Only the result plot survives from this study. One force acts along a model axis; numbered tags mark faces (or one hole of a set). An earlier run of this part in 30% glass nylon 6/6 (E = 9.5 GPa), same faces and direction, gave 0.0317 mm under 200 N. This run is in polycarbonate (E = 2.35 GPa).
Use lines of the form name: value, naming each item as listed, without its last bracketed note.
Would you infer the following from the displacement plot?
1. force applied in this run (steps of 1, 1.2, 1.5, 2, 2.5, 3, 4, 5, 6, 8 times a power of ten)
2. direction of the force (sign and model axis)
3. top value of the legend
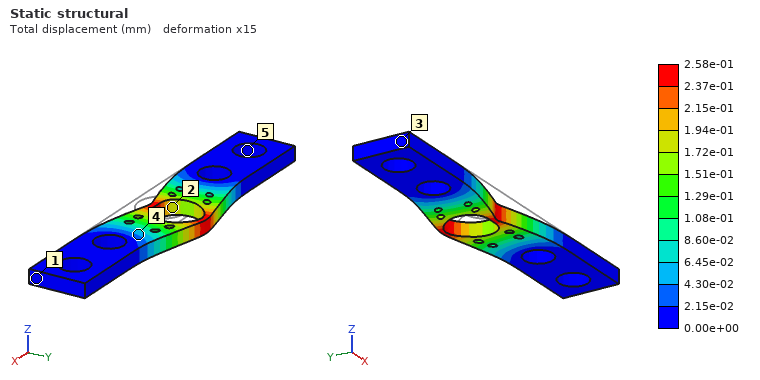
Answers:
force applied in this run: 400 N
direction of the force: +Y
top value of the legend: 2.58e-01 mm
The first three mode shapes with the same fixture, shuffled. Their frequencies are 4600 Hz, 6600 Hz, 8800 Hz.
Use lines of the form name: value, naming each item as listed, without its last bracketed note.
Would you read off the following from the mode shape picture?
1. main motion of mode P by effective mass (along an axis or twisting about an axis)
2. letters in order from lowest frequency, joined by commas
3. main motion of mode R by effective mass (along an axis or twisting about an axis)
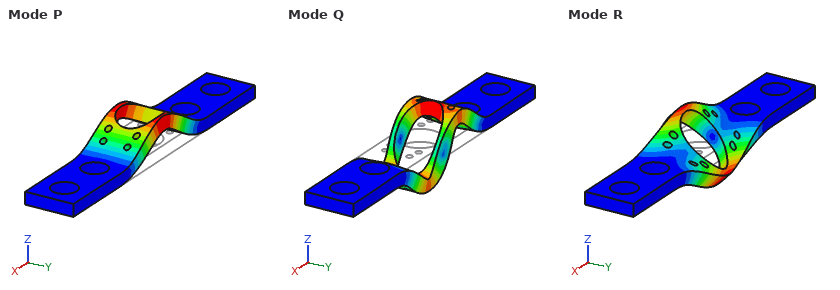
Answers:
main motion of mode P by effective mass: along Z
letters in order from lowest frequency, joined by commas: P, R, Q
main motion of mode R by effective mass: twisting about X
